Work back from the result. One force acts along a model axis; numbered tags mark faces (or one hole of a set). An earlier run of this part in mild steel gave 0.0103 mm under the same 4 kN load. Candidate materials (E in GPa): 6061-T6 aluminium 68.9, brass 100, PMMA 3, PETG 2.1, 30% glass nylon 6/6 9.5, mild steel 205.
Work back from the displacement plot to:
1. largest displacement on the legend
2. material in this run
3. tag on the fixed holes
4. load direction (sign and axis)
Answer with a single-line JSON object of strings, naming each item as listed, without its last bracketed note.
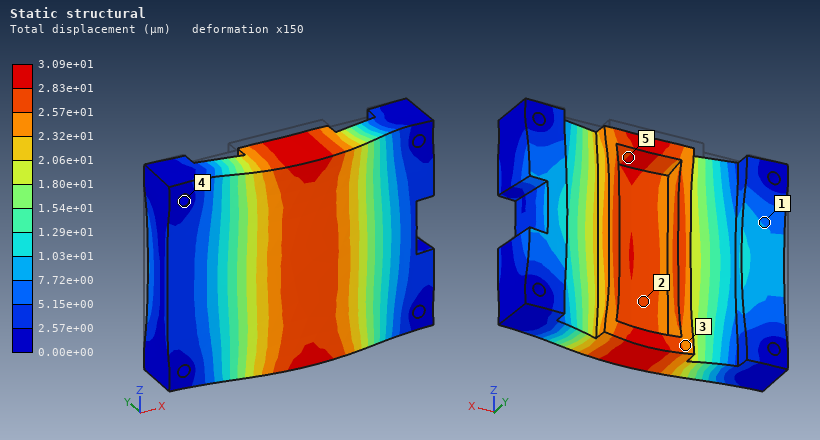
{"largest displacement on the legend": "3.09e+01 µm", "material in this run": "6061-T6 aluminium", "tag on the fixed holes": "4", "load direction": "-Y"}
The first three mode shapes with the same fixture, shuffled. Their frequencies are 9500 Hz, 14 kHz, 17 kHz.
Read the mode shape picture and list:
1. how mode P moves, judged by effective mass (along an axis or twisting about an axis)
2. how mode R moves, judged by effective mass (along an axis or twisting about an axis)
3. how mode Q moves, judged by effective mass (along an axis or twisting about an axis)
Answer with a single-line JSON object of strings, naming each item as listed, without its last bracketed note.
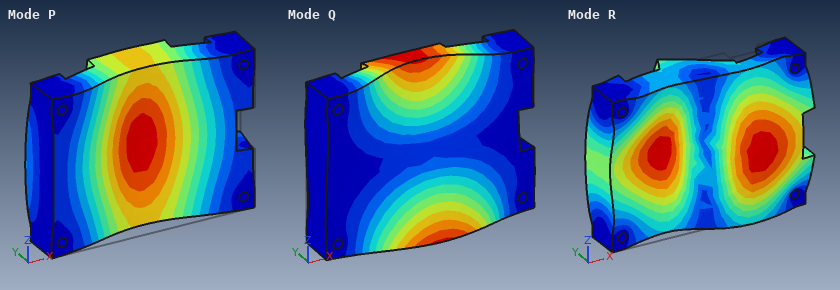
{"how mode P moves, judged by effective mass": "along Y", "how mode R moves, judged by effective mass": "twisting about Z", "how mode Q moves, judged by effective mass": "twisting about X"}
